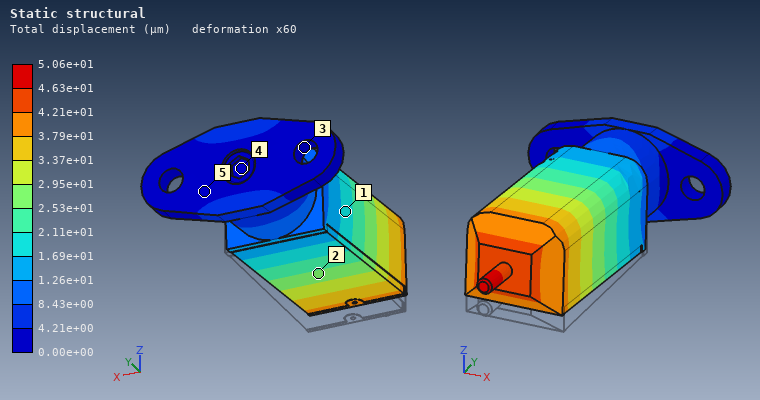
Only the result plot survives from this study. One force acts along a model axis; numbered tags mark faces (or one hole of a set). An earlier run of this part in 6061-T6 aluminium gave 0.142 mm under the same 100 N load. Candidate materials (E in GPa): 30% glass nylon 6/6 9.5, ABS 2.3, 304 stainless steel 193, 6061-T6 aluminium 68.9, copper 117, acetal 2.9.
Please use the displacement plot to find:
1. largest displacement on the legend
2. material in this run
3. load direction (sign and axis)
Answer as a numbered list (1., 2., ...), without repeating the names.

1. 5.06e+01 µm
2. 304 stainless steel
3. +Z
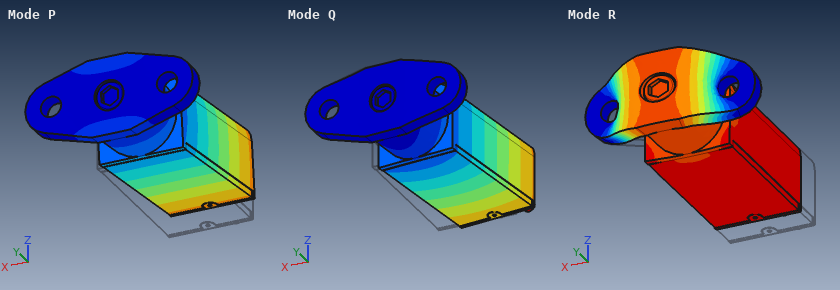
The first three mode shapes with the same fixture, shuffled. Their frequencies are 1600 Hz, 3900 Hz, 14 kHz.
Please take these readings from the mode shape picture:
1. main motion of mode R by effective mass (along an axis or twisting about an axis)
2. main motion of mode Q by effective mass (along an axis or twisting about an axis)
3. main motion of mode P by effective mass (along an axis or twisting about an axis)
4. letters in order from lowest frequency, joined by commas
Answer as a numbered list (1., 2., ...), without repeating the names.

1. along Y
2. along X
3. along Z
4. P, Q, R
